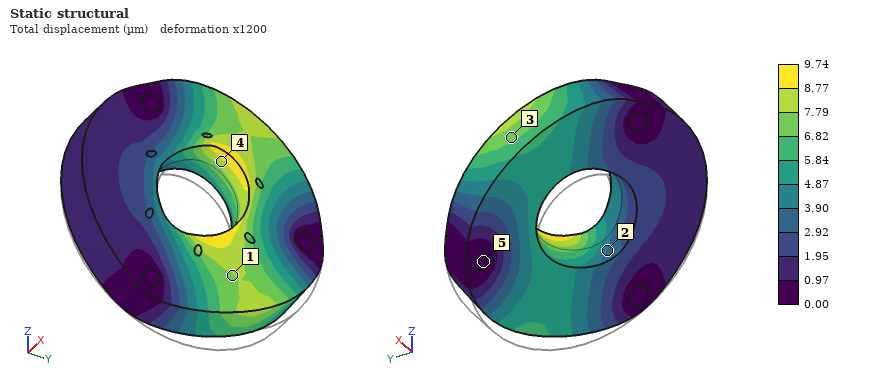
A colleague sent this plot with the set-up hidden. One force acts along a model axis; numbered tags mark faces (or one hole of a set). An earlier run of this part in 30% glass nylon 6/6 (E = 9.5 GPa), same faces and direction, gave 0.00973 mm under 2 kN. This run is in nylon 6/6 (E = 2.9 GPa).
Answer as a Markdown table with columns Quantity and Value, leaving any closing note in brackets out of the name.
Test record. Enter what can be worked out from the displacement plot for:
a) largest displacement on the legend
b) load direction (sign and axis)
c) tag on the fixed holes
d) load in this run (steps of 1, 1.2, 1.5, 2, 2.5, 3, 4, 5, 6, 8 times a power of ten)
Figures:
| Quantity | Value |
|---|---|
| largest displacement on the legend | 9.74 µm |
| load direction | +Z |
| tag on the fixed holes | 5 |
| load in this run | 600 N |
